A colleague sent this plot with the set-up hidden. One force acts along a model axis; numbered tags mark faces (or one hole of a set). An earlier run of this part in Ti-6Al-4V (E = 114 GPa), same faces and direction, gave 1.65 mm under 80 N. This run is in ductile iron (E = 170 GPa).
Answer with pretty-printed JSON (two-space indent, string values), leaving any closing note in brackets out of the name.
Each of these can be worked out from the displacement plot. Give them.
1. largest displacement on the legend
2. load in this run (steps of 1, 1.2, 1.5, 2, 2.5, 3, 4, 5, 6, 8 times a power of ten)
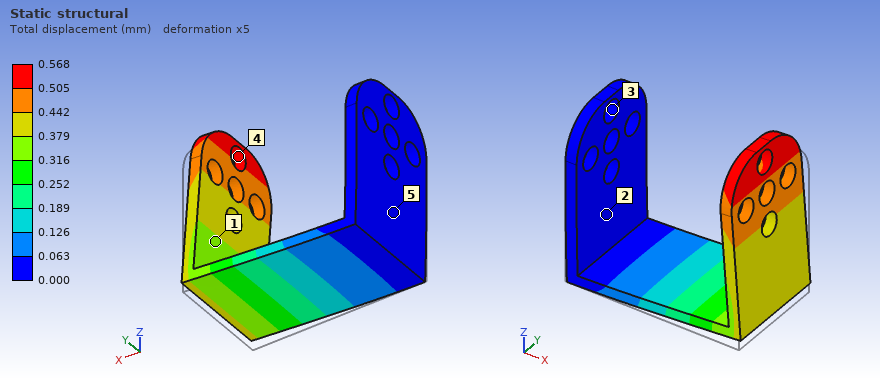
{
  "largest displacement on the legend": "0.568 mm",
  "load in this run": "40 N"
}
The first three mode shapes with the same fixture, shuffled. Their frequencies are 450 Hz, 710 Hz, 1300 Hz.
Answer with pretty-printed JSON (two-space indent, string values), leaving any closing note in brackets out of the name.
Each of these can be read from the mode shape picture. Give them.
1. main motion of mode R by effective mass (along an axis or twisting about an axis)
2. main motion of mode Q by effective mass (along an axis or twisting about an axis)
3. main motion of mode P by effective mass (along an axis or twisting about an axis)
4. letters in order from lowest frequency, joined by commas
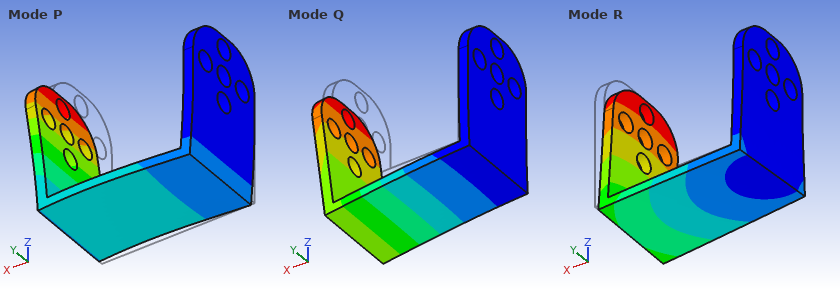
{
  "main motion of mode R by effective mass": "along Y",
  "main motion of mode Q by effective mass": "along Z",
  "main motion of mode P by effective mass": "along X",
  "letters in order from lowest frequency, joined by commas": "Q, R, P"
}
